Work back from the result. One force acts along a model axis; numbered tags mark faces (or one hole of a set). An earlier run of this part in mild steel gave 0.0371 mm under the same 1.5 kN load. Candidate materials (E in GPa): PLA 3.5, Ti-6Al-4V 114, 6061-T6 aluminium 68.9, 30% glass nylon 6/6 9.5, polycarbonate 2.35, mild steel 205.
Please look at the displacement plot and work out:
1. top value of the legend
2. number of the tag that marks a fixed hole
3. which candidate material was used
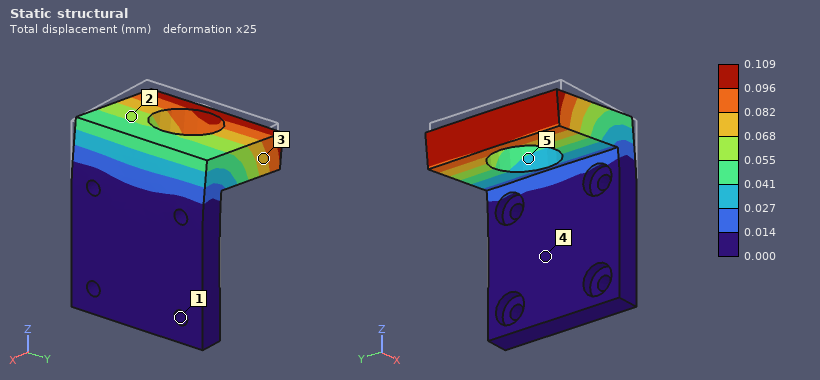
0.109 mm
1
6061-T6 aluminium
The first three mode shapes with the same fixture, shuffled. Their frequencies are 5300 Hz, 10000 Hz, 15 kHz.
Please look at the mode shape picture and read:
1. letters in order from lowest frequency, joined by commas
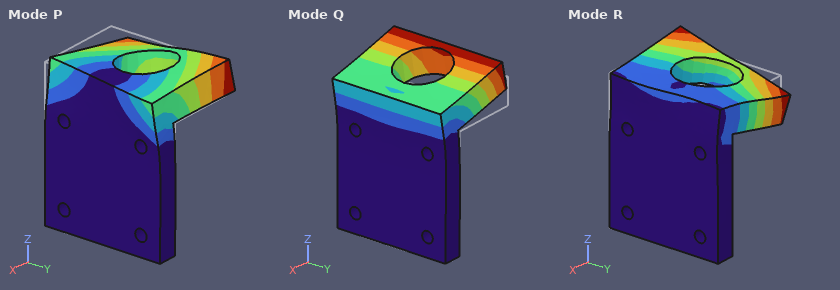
Q, P, R
